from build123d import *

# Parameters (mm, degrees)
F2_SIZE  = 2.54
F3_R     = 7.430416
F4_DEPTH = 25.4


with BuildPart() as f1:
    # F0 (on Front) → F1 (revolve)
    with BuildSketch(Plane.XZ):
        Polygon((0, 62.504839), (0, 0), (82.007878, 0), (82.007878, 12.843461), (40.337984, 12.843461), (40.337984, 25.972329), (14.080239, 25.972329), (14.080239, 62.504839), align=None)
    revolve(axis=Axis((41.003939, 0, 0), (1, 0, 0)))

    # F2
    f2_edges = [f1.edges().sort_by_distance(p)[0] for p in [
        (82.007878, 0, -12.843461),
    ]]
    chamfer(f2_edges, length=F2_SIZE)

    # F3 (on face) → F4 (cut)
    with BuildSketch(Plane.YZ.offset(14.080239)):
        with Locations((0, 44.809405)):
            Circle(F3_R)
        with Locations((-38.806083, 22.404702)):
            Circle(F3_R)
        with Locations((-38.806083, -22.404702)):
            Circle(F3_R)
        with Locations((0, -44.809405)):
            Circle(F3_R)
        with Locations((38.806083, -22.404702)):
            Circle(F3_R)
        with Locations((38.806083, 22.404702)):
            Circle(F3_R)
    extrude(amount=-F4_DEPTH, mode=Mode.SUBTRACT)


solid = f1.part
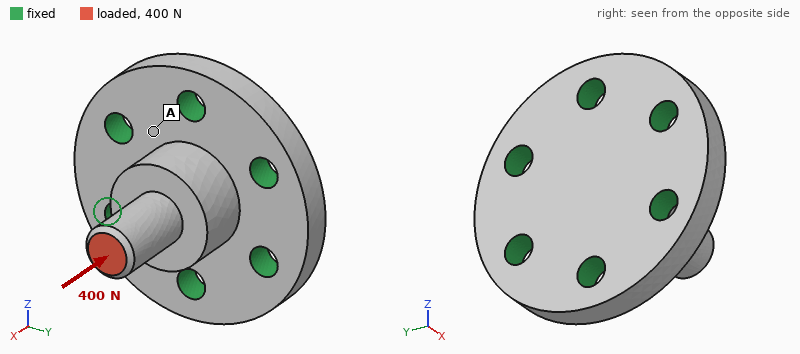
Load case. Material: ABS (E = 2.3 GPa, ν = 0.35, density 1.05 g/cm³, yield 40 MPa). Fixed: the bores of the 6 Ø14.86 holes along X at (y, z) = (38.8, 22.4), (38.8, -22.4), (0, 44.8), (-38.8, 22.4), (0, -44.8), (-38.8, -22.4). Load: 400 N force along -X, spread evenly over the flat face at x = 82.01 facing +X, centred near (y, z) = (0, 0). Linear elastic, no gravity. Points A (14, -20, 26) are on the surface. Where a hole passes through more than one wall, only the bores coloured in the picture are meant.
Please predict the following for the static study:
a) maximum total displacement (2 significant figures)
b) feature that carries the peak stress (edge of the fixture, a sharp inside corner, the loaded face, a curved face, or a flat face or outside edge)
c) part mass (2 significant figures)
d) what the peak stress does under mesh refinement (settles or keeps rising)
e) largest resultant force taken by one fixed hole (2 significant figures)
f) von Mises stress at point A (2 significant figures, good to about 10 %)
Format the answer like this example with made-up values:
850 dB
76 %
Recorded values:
26 µm
edge of the fixture
250 g
keeps rising
73 N
0.13 MPa
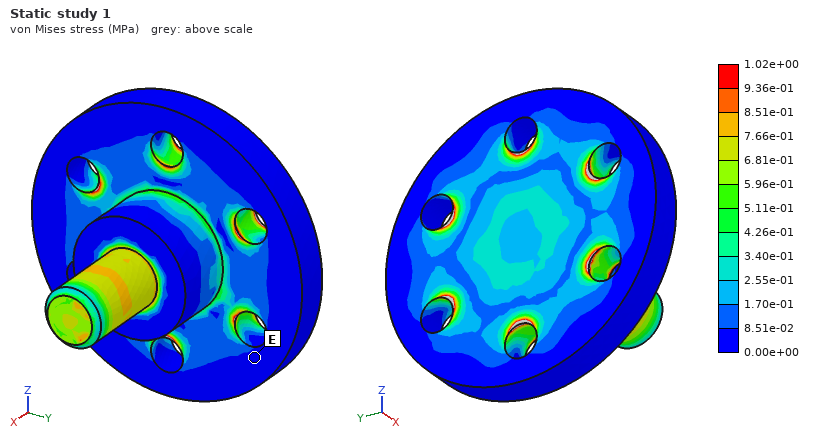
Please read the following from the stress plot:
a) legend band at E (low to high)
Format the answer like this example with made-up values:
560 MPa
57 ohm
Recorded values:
0.00e+00 to 8.51e-02 MPa
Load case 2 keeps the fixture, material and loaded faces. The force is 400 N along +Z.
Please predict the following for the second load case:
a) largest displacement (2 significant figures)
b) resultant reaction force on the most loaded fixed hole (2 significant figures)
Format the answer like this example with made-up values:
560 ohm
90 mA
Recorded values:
0.42 mm
310 N
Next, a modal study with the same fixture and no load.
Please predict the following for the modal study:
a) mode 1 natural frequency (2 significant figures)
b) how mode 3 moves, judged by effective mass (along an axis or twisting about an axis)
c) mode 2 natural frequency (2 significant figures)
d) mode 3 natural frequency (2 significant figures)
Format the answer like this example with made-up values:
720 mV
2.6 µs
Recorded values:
1700 Hz
along X
1700 Hz
3300 Hz
